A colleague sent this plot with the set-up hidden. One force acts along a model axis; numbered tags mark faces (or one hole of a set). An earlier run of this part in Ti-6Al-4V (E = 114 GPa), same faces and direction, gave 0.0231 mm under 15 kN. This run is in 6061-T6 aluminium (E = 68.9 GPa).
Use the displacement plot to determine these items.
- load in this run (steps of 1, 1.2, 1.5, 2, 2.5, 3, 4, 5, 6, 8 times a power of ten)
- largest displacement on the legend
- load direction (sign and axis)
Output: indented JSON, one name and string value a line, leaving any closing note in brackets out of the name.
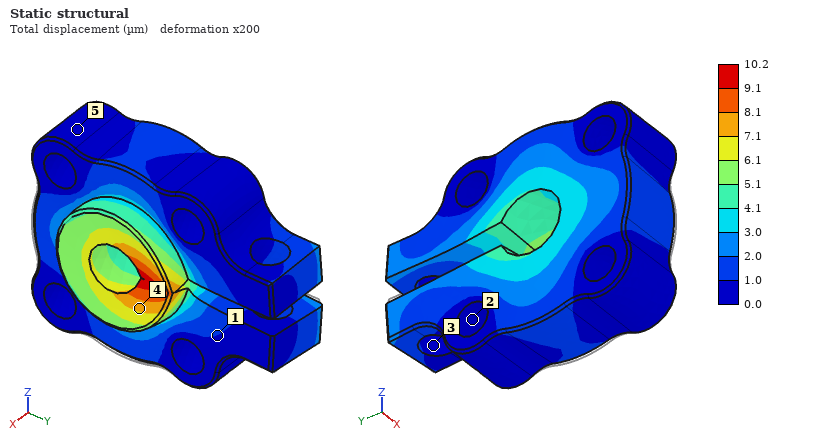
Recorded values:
{
  "load in this run": "4 kN",
  "largest displacement on the legend": "10.2 µm",
  "load direction": "-X"
}
